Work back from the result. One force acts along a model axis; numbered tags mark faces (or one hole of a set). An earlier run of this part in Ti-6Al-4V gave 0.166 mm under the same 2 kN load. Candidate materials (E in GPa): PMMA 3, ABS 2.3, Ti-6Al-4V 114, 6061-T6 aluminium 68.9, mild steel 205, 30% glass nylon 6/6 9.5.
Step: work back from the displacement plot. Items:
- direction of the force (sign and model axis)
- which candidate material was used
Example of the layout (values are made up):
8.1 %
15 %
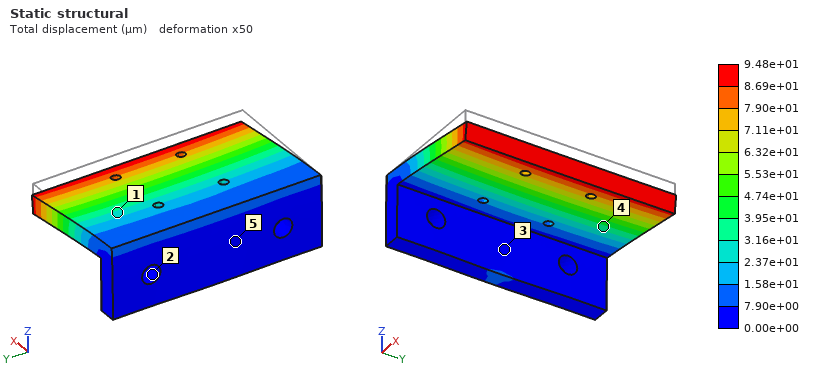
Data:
-Z
mild steel
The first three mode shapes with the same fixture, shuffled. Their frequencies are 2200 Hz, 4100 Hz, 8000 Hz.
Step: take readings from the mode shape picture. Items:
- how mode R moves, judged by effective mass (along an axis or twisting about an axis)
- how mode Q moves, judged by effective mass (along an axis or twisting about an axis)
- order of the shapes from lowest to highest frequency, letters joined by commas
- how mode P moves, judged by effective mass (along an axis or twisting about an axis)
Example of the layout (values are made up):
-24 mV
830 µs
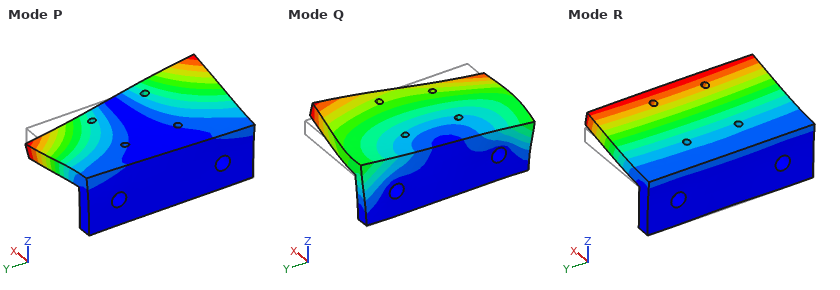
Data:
along Z
along Y
R, P, Q
twisting about X
